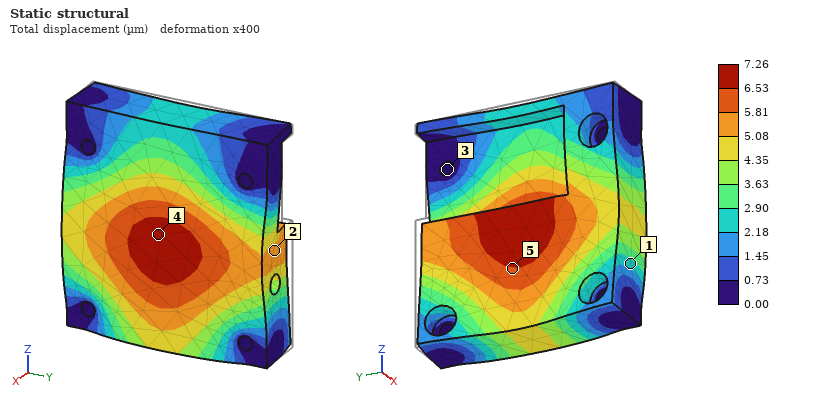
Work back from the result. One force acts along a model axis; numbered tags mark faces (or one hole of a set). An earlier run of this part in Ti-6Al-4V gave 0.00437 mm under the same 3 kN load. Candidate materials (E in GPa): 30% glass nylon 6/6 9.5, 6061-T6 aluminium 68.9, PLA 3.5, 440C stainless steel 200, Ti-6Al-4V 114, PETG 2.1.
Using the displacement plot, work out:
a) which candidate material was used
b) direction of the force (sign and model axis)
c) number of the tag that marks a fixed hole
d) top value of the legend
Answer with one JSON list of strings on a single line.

["6061-T6 aluminium", "+X", "3", "7.26 µm"]
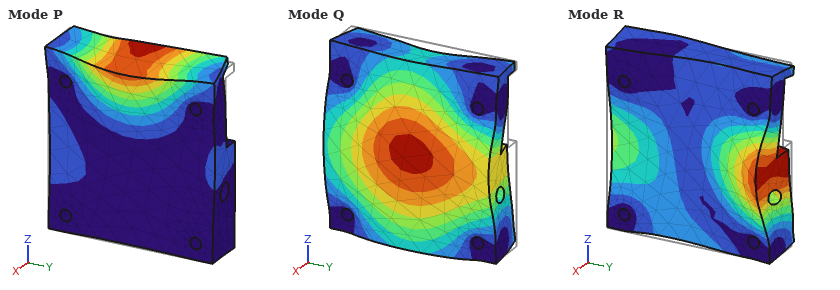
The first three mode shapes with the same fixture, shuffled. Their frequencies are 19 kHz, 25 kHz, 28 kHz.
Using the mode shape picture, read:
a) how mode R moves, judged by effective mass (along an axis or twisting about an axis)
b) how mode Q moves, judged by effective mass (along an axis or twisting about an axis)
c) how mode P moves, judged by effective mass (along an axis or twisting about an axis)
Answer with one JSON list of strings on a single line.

["twisting about Z", "along X", "twisting about Y"]
